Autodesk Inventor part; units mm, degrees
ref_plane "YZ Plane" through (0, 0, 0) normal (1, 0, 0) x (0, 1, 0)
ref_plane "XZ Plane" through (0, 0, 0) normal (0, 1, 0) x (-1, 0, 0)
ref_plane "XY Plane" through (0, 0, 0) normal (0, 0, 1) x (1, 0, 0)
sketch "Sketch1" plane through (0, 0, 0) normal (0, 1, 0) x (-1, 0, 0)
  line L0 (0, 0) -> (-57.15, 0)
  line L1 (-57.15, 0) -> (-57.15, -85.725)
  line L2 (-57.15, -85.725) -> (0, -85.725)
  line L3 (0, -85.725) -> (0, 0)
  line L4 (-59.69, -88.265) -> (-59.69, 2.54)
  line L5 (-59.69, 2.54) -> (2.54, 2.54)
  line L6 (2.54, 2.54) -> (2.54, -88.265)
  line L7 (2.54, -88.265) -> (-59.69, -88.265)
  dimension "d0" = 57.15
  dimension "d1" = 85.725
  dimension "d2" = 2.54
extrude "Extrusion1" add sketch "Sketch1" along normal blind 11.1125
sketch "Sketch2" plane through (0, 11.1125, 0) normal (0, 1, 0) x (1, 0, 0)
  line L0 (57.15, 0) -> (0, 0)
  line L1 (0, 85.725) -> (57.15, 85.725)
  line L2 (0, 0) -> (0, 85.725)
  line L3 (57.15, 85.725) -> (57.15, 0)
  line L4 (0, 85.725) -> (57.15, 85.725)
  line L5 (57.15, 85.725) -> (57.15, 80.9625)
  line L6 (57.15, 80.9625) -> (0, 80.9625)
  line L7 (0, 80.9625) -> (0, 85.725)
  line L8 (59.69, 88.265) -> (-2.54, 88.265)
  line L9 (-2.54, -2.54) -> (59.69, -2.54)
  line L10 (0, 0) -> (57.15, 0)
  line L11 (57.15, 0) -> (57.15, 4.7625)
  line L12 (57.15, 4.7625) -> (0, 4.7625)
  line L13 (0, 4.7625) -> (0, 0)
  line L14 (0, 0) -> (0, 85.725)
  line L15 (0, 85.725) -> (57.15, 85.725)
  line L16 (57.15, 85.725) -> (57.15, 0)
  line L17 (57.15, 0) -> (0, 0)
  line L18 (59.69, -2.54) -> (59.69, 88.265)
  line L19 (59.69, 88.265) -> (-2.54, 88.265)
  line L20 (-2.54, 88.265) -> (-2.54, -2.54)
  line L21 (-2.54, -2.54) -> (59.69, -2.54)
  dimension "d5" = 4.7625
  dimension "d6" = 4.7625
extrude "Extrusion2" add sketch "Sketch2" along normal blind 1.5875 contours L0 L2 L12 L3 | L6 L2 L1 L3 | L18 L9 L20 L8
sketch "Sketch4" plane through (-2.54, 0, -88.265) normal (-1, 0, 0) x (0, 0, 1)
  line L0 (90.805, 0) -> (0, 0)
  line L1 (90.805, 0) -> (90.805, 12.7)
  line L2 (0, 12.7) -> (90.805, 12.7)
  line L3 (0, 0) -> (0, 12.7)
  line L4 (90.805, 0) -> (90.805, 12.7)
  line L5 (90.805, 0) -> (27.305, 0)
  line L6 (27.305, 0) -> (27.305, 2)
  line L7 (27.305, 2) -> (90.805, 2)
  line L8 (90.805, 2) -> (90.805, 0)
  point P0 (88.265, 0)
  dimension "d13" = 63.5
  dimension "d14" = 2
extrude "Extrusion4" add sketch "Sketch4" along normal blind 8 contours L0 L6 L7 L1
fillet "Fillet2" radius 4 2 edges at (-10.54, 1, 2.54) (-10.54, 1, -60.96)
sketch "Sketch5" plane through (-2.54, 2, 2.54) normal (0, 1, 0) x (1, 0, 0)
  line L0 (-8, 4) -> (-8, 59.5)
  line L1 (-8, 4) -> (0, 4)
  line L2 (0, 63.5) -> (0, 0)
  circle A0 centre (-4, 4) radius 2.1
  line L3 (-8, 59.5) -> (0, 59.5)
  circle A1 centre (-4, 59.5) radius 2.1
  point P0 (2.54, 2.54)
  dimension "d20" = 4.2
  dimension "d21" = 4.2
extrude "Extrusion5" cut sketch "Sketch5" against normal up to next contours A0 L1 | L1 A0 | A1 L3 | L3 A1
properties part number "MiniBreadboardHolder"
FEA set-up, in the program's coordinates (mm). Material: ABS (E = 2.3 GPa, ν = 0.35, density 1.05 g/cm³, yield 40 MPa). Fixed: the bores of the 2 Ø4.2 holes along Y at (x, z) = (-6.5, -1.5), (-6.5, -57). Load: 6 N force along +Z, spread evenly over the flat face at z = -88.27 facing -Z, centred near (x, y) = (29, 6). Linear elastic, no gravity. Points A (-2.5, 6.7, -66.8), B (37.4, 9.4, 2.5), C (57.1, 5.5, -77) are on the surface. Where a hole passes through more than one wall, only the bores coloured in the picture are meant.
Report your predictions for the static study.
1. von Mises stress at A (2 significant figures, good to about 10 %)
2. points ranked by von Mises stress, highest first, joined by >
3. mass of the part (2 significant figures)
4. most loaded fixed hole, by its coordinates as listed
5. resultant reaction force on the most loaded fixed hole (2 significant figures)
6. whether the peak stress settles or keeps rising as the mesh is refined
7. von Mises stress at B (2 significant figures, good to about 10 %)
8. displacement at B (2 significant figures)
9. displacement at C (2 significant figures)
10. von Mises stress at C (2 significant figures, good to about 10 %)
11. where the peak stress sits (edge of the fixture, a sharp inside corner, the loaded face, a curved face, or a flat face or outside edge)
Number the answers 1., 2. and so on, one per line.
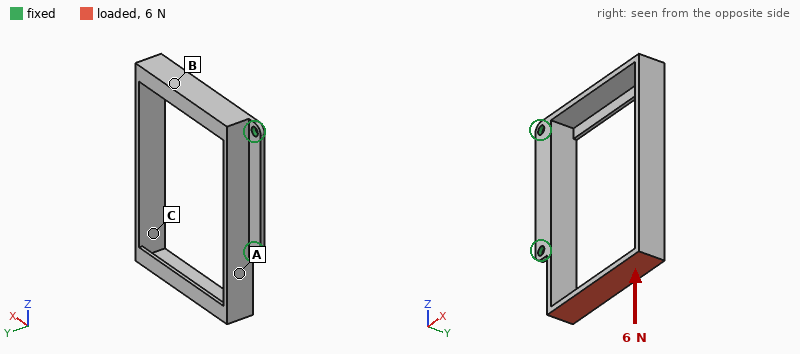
1. 2.3 MPa
2. A > C > B
3. 12 g
4. (-6.5, -57)
5. 4.8 N
6. keeps rising
7. 0.55 MPa
8. 0.68 mm
9. 1.1 mm
10. 1.5 MPa
11. a sharp inside corner
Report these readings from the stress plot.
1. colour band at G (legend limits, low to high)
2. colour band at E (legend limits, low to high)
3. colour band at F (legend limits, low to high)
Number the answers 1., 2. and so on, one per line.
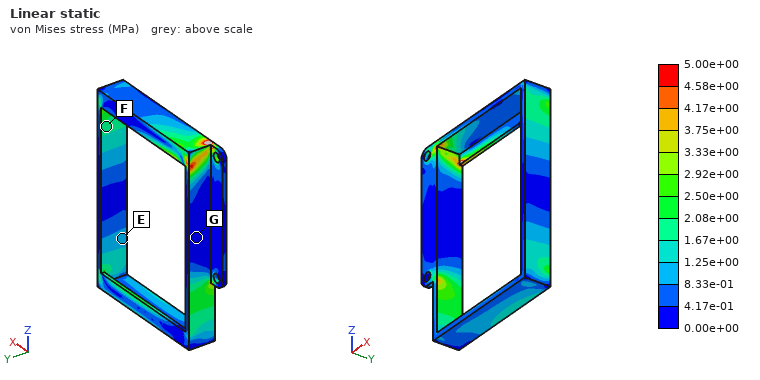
1. 0.00e+00 to 4.17e-01 MPa
2. 8.33e-01 to 1.25e+00 MPa
3. 1.67e+00 to 2.08e+00 MPa
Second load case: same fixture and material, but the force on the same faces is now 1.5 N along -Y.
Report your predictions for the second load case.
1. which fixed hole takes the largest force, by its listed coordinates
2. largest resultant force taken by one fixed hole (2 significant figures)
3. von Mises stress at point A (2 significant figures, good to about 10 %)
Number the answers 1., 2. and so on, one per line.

1. (-6.5, -57)
2. 2.8 N
3. 1.6 MPa
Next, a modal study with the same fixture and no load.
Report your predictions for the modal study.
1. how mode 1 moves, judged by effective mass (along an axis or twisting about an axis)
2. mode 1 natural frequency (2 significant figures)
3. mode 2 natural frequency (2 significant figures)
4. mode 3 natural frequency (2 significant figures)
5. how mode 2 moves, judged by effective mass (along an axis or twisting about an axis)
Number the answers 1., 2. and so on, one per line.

1. along Y
2. 85 Hz
3. 120 Hz
4. 200 Hz
5. along Z
